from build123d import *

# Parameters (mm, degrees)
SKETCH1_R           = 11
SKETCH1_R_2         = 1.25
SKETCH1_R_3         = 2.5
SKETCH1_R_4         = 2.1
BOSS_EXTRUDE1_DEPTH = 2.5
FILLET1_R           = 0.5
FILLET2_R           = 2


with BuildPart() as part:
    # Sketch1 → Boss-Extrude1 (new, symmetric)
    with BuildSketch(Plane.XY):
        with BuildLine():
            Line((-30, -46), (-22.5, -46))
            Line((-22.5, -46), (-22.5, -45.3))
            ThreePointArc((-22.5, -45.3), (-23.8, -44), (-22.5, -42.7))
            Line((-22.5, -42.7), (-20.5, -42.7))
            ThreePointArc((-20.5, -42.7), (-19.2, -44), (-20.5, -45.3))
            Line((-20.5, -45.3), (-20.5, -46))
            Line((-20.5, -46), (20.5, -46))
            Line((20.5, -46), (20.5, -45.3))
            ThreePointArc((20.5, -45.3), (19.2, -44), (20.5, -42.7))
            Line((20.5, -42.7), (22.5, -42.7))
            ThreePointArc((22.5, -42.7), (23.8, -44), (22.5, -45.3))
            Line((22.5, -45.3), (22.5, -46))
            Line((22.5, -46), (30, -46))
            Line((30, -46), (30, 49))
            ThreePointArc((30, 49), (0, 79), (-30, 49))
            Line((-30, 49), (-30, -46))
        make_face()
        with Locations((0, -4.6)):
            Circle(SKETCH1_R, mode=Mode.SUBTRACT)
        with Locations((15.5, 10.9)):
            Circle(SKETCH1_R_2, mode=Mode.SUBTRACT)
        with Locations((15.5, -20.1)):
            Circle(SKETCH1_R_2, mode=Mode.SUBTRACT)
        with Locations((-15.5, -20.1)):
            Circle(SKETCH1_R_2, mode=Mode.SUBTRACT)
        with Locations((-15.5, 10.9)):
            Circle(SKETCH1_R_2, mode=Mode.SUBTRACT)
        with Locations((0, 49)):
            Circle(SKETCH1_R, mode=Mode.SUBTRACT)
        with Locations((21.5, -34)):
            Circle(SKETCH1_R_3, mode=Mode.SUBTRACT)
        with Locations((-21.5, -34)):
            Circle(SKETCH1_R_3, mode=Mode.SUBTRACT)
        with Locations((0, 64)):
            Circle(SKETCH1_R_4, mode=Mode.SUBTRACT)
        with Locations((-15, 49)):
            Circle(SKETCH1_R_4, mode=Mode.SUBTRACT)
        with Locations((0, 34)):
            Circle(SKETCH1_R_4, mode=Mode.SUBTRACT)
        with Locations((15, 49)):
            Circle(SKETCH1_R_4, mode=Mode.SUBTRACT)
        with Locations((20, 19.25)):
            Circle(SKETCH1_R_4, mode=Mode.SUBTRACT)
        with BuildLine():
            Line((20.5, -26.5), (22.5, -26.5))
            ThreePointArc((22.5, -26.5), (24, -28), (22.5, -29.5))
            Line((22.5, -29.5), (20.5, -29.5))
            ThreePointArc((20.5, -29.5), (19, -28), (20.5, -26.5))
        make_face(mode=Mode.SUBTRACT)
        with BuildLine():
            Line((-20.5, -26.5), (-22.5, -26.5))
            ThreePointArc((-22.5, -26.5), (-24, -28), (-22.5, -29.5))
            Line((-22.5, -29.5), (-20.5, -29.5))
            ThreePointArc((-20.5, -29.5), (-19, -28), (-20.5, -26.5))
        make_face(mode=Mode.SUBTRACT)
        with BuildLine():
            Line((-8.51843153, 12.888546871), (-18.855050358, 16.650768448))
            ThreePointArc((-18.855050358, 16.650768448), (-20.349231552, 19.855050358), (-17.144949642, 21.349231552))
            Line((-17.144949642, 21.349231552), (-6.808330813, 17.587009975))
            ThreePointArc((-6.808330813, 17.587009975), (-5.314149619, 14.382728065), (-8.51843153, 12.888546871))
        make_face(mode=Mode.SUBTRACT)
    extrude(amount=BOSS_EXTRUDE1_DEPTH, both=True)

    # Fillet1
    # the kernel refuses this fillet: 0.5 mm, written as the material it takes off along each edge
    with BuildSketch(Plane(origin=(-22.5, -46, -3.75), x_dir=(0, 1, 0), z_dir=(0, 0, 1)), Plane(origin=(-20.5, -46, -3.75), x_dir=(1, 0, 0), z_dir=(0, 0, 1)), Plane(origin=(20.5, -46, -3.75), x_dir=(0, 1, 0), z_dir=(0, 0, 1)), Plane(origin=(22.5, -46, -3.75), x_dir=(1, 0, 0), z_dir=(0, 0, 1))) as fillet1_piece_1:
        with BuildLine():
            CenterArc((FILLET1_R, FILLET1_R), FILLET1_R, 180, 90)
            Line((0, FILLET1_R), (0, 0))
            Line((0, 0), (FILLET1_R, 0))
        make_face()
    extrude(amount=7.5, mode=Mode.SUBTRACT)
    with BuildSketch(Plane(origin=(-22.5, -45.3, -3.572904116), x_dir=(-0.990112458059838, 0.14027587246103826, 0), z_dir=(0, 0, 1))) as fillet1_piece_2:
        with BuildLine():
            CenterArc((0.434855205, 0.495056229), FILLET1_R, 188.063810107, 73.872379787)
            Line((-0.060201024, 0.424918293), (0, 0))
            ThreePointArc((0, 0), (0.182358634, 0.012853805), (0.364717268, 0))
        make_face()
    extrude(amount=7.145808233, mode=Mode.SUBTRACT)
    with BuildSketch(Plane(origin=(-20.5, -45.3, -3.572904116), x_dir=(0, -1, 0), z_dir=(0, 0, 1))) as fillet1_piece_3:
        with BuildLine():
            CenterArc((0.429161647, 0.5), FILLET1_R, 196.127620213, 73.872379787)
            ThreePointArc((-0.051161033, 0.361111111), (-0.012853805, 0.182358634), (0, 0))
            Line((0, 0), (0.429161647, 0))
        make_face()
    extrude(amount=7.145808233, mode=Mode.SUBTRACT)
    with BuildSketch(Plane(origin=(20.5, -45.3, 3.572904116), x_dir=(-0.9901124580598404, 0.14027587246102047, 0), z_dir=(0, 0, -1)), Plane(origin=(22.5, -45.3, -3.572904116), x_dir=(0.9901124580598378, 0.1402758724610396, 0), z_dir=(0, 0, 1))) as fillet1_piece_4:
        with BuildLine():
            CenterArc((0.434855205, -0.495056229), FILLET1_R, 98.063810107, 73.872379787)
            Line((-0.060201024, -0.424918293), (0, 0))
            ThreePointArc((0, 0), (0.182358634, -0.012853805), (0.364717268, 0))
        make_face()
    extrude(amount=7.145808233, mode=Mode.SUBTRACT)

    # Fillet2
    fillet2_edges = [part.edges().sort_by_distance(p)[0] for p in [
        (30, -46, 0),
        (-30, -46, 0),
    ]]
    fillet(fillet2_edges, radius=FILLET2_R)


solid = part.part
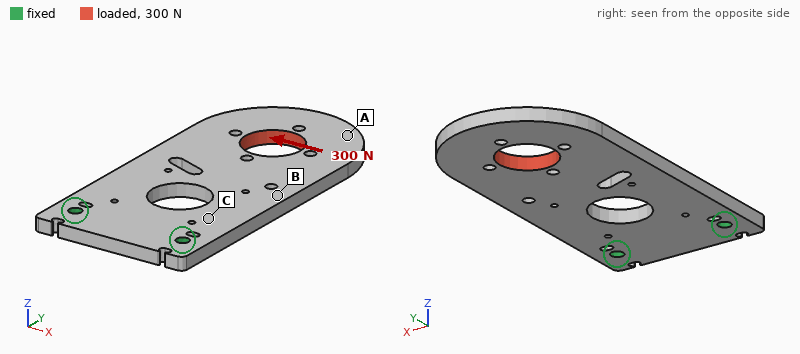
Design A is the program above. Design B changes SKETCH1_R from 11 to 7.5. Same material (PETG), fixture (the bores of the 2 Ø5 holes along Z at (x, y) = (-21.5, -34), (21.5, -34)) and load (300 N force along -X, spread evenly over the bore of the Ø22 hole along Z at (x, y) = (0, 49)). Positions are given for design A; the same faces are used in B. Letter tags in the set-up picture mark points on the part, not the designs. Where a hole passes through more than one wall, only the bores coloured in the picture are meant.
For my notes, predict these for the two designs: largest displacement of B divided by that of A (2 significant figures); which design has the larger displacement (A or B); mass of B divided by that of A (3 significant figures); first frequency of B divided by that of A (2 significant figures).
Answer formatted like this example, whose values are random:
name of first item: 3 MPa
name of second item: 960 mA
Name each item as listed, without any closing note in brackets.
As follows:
largest displacement of B divided by that of A: 0.90
which design has the larger displacement: A
mass of B divided by that of A: 1.07
first frequency of B divided by that of A: 1.0
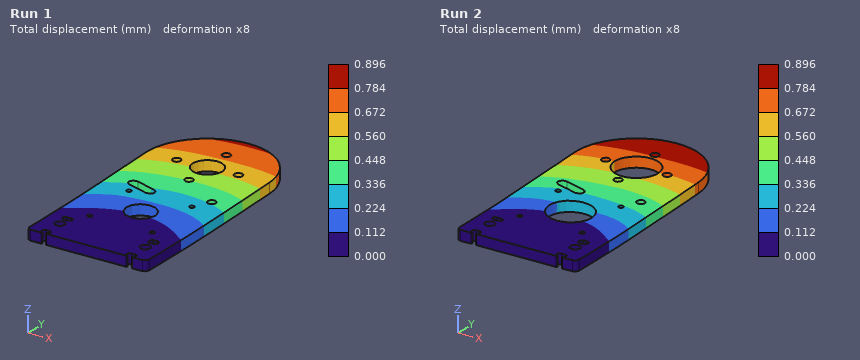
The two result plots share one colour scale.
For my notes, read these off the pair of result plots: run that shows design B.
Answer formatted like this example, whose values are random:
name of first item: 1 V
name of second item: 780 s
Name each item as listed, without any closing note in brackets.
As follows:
run that shows design B: Run 1
